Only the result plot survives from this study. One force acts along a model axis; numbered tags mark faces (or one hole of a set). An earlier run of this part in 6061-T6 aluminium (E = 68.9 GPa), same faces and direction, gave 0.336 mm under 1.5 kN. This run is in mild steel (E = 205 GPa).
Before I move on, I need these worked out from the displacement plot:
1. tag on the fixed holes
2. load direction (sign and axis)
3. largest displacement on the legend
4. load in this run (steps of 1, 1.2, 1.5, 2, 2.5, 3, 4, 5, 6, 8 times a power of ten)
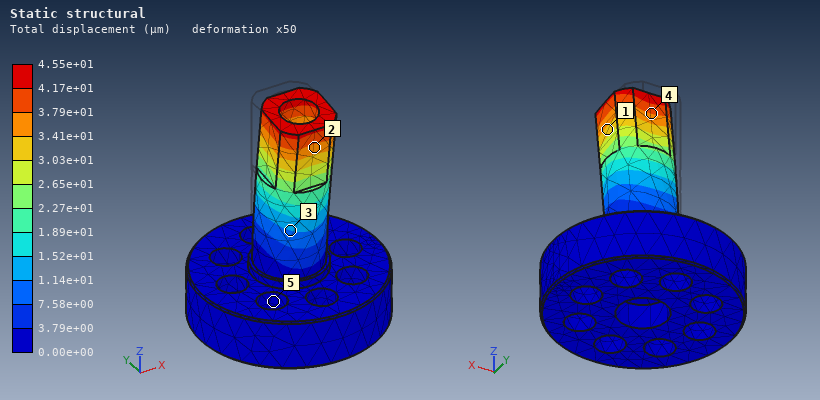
5
-Y
4.55e+01 µm
600 N
